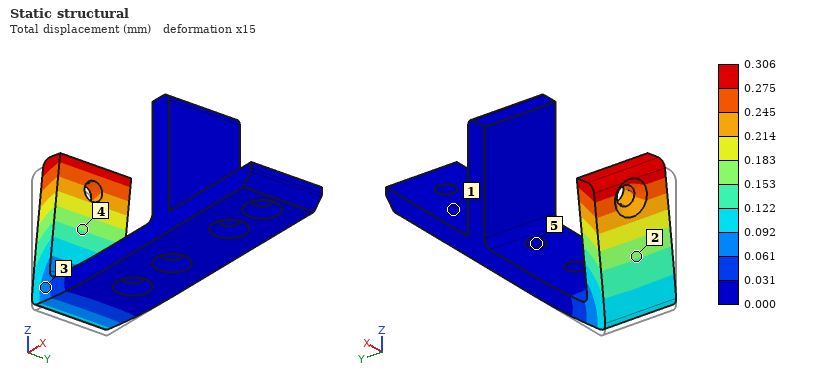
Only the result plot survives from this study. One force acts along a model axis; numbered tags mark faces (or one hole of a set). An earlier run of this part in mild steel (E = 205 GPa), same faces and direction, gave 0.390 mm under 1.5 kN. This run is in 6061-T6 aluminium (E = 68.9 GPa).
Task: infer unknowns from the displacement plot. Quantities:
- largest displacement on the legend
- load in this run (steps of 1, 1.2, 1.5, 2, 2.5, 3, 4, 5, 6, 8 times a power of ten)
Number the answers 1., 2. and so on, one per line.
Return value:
1. 0.306 mm
2. 400 N
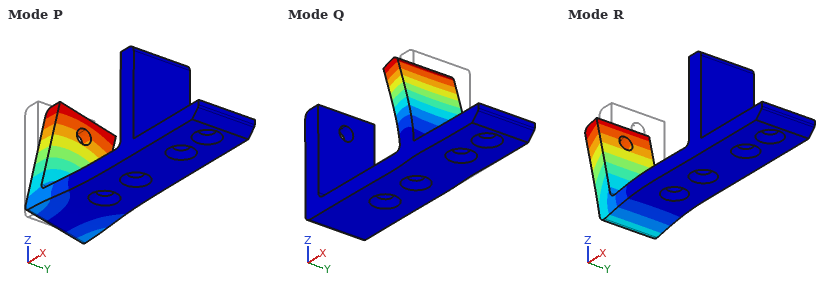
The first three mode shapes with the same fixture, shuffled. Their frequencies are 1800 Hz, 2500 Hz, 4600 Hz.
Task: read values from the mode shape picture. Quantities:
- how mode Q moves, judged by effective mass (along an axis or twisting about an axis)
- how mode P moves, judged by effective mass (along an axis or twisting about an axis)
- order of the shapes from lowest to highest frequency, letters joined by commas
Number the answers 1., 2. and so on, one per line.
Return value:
1. along X
2. along Y
3. R, P, Q
